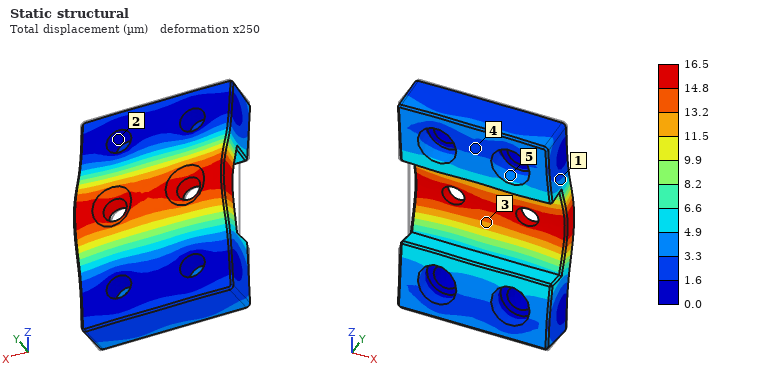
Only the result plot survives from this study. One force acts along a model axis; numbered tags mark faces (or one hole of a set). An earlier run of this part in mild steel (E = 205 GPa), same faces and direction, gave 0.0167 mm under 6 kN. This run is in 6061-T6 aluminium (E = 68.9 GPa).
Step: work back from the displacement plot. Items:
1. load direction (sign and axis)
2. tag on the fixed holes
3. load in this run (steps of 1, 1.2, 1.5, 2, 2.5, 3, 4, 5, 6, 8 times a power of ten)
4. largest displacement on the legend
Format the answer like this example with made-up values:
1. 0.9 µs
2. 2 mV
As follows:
1. +Y
2. 2
3. 2 kN
4. 16.5 µm
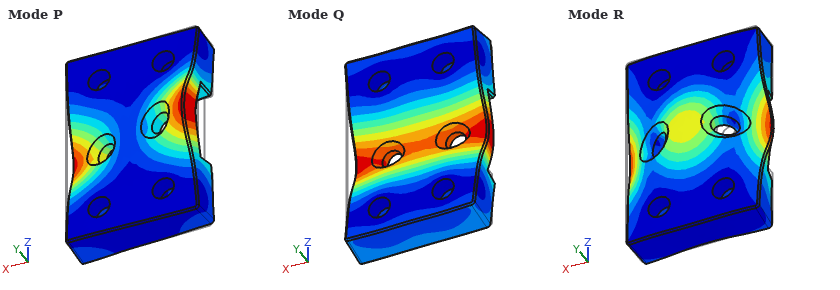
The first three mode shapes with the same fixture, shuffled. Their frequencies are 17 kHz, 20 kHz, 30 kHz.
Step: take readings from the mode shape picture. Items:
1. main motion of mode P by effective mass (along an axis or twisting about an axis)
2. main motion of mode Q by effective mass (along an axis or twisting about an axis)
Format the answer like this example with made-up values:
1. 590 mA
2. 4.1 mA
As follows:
1. twisting about Z
2. along Y
